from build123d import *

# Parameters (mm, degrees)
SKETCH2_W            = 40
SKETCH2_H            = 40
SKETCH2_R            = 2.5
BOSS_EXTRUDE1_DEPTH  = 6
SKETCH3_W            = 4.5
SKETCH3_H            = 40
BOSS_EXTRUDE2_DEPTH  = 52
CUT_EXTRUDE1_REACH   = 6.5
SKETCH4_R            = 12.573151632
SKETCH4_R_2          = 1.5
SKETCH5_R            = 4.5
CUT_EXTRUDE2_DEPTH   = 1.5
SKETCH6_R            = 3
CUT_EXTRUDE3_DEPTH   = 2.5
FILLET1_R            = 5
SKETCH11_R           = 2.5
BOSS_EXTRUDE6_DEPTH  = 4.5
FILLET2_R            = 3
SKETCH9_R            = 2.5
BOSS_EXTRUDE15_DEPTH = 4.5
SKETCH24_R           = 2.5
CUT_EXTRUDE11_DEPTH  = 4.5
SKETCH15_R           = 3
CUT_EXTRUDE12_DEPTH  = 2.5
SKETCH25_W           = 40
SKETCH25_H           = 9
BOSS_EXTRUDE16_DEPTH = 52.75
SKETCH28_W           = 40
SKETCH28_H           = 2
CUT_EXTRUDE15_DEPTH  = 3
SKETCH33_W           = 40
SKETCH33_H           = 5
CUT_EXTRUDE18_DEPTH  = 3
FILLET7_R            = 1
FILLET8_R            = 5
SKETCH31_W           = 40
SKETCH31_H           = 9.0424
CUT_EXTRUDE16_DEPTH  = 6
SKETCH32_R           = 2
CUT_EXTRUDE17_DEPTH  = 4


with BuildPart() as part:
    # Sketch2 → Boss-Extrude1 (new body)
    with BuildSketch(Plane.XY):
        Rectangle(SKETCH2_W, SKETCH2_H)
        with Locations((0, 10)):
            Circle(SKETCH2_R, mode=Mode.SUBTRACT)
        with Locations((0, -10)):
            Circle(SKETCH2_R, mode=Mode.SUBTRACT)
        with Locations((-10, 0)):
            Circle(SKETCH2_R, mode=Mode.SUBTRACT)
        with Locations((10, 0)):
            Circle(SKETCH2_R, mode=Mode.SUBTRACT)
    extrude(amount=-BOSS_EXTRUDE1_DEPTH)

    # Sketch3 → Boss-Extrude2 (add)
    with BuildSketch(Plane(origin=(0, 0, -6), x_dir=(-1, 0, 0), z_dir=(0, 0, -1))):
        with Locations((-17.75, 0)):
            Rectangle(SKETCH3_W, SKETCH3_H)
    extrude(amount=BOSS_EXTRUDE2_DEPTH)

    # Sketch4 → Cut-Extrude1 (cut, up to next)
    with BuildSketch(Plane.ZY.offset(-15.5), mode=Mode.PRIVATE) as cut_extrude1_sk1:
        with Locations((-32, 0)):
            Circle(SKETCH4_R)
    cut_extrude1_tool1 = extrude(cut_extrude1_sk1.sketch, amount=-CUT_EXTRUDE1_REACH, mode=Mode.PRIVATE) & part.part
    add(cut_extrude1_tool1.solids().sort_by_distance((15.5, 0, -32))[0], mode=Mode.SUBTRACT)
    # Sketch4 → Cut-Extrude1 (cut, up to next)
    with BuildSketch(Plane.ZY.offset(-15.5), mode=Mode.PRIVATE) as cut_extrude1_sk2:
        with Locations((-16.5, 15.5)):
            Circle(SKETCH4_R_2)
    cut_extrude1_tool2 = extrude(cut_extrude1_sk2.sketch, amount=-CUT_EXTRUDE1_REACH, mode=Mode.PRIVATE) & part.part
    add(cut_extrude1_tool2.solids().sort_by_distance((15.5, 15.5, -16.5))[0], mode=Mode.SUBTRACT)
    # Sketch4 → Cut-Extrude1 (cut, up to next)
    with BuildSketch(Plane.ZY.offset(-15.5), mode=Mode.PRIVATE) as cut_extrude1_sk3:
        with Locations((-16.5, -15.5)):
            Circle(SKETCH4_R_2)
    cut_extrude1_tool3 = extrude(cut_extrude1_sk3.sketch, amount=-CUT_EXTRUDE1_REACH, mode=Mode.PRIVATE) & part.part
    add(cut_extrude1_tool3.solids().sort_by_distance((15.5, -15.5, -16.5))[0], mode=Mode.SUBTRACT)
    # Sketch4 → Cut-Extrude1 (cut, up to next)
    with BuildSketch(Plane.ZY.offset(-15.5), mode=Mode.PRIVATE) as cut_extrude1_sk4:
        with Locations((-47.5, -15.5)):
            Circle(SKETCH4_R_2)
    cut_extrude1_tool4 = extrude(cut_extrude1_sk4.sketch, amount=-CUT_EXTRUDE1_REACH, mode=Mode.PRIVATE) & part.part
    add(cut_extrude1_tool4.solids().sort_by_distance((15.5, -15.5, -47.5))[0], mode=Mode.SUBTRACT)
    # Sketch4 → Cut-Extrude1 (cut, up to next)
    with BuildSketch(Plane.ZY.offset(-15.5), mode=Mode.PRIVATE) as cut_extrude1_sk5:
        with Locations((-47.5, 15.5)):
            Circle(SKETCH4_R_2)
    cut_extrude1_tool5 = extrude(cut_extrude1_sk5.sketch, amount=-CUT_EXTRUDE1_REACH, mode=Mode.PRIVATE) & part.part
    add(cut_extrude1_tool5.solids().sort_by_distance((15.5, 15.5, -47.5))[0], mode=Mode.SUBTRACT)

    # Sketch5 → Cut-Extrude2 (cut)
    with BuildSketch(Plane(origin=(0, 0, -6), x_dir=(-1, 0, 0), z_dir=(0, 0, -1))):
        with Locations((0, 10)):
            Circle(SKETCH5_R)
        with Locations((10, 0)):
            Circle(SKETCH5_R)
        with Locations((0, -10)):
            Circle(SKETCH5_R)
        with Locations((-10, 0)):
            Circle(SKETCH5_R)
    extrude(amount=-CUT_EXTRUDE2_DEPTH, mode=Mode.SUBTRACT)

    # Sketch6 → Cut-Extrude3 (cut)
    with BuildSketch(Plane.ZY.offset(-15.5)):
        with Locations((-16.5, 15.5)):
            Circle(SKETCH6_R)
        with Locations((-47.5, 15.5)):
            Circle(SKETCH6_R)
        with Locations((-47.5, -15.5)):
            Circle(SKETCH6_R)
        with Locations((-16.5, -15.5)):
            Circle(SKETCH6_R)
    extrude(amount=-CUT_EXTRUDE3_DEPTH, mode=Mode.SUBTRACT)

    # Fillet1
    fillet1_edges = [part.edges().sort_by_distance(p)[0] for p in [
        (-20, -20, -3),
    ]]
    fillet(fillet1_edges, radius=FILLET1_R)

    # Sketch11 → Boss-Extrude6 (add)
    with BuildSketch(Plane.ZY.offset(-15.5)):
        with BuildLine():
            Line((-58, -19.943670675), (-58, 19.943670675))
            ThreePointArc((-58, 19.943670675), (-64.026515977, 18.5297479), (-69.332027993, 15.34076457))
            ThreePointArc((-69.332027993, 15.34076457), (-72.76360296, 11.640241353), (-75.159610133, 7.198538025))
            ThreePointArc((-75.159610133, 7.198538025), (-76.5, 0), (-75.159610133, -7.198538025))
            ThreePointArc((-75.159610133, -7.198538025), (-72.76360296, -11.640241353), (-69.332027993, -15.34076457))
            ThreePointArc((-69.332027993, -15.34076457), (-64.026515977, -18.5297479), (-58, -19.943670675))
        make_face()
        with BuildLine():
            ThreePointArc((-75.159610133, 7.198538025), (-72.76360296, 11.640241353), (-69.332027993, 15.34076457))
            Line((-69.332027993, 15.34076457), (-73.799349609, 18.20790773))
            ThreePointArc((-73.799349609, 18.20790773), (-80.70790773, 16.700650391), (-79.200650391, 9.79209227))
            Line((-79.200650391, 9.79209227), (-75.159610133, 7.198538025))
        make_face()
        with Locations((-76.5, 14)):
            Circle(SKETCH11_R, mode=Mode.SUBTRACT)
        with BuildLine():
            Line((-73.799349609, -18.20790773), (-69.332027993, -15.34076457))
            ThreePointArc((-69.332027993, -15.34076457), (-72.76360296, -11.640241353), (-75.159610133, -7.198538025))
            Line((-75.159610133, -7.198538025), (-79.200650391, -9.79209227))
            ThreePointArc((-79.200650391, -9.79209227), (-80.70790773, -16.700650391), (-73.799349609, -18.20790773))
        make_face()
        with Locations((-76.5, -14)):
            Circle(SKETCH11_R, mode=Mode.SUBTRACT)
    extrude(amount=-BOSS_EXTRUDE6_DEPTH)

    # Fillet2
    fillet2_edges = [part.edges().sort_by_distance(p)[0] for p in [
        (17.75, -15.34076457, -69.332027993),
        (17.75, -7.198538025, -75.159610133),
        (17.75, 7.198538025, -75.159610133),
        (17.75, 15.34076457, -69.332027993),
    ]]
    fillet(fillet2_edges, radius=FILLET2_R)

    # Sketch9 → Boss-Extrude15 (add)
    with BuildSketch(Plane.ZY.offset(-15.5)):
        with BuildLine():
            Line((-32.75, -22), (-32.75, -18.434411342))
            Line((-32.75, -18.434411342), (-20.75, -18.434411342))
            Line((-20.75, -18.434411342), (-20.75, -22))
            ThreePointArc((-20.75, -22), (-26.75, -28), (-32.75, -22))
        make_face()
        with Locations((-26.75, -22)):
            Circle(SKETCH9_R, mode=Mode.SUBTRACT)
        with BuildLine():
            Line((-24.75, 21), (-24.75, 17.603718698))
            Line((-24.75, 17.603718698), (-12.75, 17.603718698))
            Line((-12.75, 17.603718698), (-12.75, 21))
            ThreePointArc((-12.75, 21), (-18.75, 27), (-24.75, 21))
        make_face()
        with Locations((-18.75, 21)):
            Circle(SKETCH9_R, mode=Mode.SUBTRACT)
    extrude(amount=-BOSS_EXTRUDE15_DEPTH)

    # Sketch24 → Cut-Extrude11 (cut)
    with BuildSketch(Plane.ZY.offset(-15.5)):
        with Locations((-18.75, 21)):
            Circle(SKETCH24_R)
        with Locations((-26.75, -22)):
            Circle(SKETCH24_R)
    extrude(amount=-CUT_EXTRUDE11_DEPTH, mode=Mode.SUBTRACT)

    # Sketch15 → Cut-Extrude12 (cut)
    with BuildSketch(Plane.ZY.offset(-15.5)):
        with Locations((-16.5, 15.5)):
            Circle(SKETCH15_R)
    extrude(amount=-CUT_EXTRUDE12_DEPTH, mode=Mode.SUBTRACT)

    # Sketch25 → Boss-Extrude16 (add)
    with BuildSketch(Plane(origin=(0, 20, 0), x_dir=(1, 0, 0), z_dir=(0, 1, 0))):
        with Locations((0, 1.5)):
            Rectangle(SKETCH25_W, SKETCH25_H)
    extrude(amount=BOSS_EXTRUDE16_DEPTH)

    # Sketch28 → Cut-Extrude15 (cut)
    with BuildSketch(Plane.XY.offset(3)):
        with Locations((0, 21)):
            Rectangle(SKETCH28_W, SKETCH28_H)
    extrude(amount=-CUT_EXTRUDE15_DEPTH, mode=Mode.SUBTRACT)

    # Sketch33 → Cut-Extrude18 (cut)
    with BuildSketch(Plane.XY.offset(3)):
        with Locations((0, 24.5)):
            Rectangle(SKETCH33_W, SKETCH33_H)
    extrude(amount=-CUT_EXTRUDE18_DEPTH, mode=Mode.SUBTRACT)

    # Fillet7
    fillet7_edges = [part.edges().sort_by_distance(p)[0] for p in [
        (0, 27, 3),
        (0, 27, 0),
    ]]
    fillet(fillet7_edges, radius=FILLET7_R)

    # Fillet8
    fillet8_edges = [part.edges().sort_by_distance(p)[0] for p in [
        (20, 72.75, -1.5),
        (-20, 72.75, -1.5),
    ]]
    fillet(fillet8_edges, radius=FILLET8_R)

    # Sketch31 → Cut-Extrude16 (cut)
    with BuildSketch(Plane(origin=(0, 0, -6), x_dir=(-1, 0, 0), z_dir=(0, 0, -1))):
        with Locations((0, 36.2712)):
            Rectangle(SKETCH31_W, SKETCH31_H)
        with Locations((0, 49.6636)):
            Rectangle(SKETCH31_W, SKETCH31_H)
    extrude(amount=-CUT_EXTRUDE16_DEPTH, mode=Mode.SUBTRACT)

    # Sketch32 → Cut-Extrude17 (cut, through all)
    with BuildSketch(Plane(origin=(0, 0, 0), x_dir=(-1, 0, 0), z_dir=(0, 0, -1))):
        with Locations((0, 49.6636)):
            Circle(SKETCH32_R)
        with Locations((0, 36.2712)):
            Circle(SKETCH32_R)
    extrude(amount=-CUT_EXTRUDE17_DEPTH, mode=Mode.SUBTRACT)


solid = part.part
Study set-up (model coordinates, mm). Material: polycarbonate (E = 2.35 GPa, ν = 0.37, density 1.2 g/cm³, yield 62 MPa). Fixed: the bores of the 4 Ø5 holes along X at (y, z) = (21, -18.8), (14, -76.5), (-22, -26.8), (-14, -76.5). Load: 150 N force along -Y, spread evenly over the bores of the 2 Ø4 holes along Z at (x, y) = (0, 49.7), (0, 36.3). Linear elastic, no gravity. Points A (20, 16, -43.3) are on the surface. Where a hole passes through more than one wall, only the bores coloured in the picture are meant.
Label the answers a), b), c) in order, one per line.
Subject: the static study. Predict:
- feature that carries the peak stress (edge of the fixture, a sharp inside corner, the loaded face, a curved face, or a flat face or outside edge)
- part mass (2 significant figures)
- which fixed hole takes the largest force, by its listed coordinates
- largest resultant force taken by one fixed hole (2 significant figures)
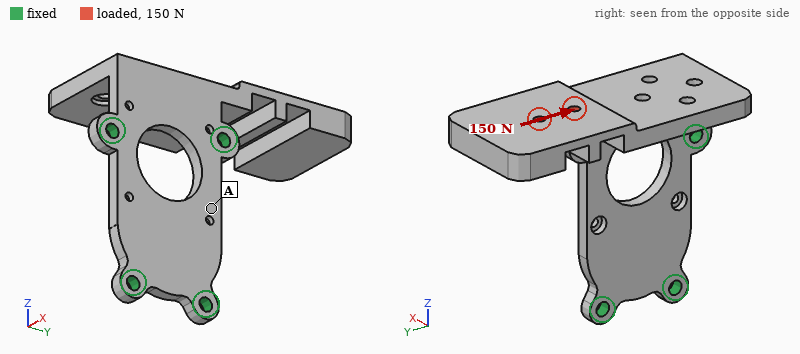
a) a flat face or outside edge
b) 40 g
c) (21, -18.8)
d) 140 N
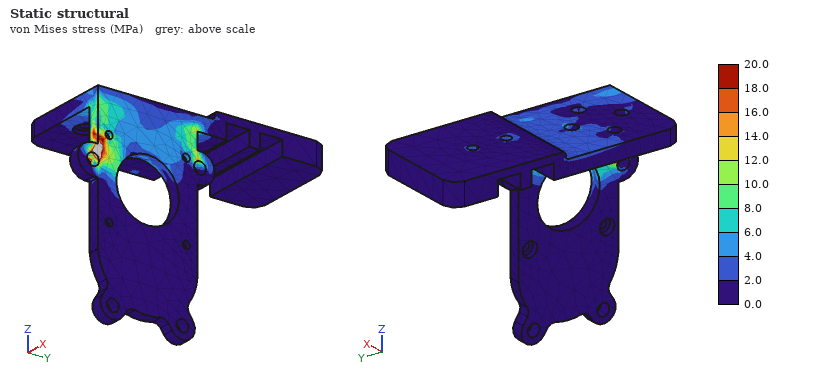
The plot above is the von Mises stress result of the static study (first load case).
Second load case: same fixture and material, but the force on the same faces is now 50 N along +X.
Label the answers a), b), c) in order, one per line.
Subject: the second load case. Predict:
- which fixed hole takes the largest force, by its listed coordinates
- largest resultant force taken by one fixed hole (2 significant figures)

a) (21, -18.8)
b) 86 N
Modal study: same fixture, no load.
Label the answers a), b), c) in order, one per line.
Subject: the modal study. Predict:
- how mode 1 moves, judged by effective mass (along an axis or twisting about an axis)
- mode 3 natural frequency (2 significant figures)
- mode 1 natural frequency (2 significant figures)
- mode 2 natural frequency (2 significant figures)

a) along Z
b) 270 Hz
c) 160 Hz
d) 270 Hz
